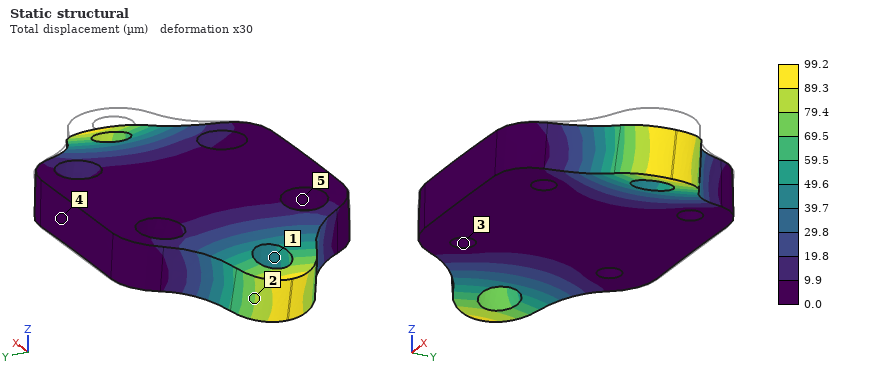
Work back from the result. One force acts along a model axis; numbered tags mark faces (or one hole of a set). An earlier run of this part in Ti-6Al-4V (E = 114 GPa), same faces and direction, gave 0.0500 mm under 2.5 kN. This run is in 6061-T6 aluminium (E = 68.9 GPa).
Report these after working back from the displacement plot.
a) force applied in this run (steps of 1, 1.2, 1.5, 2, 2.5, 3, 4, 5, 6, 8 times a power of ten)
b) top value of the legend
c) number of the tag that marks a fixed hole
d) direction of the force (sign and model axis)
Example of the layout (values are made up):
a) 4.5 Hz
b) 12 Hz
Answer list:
a) 3 kN
b) 99.2 µm
c) 3
d) -Z
